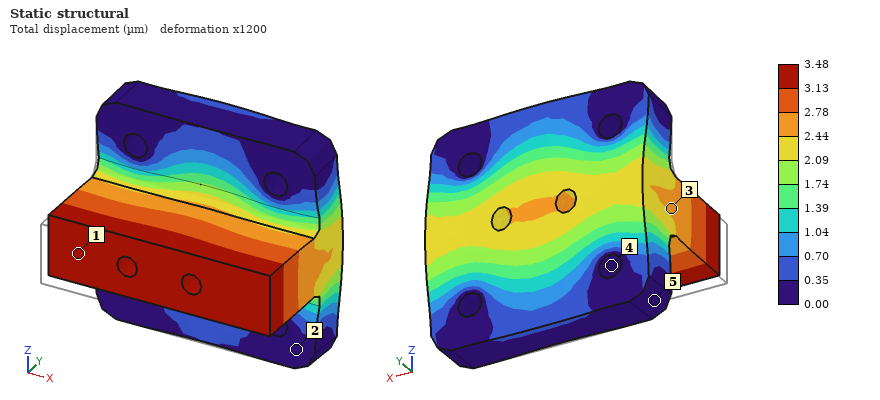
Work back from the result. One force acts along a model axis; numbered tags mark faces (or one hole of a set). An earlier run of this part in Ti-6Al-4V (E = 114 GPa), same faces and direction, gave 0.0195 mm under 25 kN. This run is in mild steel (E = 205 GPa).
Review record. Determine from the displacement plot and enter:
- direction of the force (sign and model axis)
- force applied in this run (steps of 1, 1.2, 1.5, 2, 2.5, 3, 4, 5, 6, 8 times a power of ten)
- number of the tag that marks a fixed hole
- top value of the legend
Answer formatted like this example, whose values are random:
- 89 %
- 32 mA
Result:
- +Y
- 8 kN
- 4
- 3.48 µm
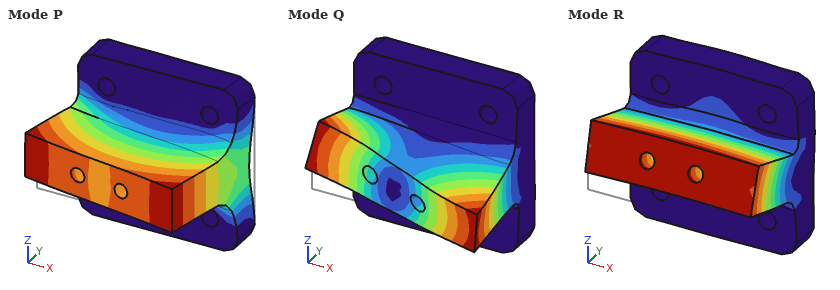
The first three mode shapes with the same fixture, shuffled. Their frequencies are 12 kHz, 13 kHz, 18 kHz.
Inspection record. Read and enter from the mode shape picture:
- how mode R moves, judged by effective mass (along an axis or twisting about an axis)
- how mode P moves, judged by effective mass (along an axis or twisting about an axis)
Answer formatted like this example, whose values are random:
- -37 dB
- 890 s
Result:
- along Z
- along X
